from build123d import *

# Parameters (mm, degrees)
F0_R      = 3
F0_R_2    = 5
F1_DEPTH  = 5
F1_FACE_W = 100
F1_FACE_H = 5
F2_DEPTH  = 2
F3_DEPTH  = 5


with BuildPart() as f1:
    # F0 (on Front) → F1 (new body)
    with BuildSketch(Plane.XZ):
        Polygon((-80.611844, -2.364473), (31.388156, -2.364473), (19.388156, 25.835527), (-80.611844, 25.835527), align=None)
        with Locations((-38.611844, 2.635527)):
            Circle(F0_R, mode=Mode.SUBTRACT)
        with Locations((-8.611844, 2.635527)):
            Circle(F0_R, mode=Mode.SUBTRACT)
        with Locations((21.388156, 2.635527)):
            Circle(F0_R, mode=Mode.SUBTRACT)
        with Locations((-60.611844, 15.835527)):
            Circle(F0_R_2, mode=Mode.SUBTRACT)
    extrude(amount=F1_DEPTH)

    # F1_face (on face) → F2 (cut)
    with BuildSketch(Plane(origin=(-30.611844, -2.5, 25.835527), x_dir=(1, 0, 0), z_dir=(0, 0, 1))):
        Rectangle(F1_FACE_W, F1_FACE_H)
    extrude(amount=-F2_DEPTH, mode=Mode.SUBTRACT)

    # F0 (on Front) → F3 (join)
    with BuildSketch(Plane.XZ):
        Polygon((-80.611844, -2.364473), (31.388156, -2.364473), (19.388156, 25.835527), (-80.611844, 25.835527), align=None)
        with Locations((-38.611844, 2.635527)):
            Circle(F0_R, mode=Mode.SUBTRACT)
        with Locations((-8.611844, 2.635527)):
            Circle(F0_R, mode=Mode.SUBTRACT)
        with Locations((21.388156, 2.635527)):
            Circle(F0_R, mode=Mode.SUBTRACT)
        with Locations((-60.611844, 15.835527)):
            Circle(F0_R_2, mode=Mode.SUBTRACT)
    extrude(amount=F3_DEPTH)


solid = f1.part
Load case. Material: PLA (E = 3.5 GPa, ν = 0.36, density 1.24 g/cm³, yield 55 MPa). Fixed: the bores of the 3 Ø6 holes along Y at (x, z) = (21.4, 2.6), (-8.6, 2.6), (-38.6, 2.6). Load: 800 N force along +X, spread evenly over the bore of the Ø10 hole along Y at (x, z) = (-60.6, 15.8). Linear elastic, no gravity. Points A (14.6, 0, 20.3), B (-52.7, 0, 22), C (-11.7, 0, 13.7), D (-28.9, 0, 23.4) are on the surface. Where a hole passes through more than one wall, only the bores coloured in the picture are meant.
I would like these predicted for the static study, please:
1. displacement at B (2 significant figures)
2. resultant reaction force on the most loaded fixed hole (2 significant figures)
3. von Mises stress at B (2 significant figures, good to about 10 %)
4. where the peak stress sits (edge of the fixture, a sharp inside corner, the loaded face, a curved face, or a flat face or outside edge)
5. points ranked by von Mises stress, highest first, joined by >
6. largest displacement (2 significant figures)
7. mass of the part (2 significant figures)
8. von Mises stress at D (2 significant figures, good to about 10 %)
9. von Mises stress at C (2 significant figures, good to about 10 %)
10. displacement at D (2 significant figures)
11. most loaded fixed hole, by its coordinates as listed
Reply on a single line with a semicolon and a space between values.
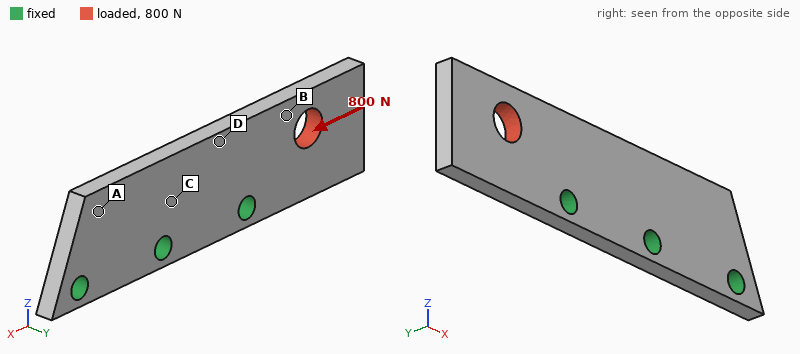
0.12 mm; 490 N; 10 MPa; edge of the fixture; B > D > C > A; 0.27 mm; 18 g; 7.4 MPa; 3.4 MPa; 0.047 mm; (-38.6, 2.6)
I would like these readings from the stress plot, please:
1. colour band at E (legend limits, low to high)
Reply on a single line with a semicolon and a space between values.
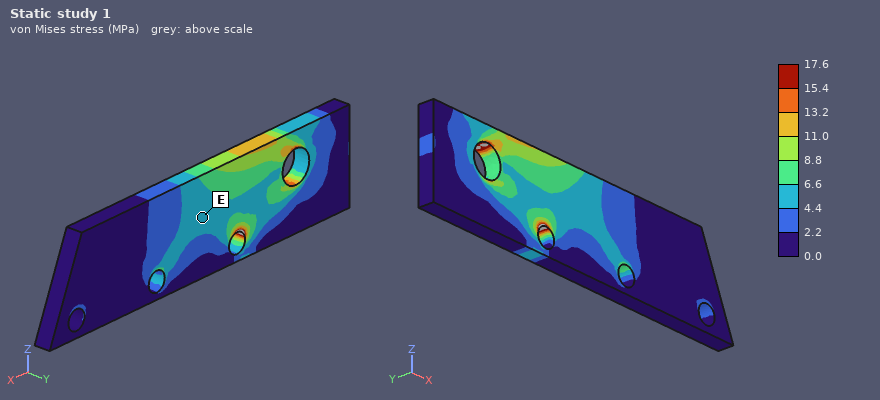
4.4 to 6.6 MPa
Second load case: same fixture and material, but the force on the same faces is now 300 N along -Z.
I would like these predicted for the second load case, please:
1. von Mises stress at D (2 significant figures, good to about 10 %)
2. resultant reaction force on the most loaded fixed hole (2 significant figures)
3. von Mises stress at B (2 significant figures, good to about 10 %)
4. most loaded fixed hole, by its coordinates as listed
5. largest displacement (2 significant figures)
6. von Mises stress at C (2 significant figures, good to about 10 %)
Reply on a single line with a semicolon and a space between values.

4.8 MPa; 460 N; 2.7 MPa; (-38.6, 2.6); 0.23 mm; 1.9 MPa
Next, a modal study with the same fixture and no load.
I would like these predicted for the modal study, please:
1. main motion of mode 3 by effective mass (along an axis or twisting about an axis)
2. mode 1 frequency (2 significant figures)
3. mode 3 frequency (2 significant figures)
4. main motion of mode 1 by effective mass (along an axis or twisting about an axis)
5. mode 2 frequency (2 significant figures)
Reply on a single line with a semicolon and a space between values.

along Z; 720 Hz; 2500 Hz; along Y; 1800 Hz
